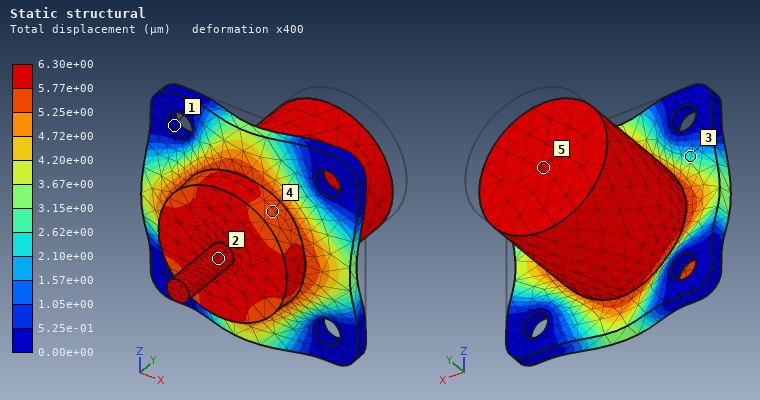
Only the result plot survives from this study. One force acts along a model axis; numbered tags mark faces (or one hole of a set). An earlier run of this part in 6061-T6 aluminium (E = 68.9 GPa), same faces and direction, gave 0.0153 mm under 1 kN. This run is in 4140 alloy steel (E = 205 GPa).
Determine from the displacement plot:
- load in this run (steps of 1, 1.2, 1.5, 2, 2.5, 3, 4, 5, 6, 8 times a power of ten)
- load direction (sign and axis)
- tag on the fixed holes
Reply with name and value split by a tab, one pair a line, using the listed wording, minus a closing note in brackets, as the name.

load in this run	1.2 kN
load direction	-Y
tag on the fixed holes	1
